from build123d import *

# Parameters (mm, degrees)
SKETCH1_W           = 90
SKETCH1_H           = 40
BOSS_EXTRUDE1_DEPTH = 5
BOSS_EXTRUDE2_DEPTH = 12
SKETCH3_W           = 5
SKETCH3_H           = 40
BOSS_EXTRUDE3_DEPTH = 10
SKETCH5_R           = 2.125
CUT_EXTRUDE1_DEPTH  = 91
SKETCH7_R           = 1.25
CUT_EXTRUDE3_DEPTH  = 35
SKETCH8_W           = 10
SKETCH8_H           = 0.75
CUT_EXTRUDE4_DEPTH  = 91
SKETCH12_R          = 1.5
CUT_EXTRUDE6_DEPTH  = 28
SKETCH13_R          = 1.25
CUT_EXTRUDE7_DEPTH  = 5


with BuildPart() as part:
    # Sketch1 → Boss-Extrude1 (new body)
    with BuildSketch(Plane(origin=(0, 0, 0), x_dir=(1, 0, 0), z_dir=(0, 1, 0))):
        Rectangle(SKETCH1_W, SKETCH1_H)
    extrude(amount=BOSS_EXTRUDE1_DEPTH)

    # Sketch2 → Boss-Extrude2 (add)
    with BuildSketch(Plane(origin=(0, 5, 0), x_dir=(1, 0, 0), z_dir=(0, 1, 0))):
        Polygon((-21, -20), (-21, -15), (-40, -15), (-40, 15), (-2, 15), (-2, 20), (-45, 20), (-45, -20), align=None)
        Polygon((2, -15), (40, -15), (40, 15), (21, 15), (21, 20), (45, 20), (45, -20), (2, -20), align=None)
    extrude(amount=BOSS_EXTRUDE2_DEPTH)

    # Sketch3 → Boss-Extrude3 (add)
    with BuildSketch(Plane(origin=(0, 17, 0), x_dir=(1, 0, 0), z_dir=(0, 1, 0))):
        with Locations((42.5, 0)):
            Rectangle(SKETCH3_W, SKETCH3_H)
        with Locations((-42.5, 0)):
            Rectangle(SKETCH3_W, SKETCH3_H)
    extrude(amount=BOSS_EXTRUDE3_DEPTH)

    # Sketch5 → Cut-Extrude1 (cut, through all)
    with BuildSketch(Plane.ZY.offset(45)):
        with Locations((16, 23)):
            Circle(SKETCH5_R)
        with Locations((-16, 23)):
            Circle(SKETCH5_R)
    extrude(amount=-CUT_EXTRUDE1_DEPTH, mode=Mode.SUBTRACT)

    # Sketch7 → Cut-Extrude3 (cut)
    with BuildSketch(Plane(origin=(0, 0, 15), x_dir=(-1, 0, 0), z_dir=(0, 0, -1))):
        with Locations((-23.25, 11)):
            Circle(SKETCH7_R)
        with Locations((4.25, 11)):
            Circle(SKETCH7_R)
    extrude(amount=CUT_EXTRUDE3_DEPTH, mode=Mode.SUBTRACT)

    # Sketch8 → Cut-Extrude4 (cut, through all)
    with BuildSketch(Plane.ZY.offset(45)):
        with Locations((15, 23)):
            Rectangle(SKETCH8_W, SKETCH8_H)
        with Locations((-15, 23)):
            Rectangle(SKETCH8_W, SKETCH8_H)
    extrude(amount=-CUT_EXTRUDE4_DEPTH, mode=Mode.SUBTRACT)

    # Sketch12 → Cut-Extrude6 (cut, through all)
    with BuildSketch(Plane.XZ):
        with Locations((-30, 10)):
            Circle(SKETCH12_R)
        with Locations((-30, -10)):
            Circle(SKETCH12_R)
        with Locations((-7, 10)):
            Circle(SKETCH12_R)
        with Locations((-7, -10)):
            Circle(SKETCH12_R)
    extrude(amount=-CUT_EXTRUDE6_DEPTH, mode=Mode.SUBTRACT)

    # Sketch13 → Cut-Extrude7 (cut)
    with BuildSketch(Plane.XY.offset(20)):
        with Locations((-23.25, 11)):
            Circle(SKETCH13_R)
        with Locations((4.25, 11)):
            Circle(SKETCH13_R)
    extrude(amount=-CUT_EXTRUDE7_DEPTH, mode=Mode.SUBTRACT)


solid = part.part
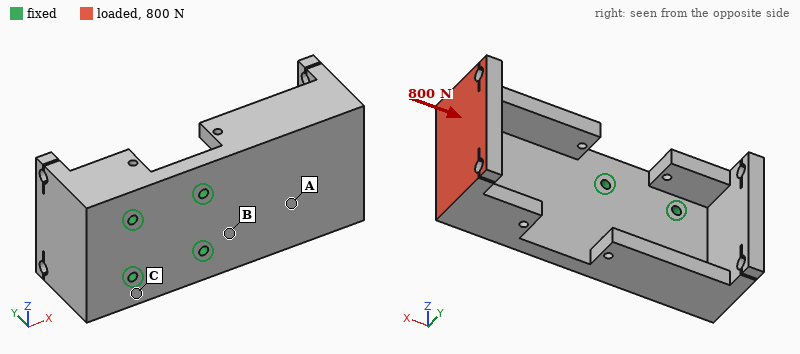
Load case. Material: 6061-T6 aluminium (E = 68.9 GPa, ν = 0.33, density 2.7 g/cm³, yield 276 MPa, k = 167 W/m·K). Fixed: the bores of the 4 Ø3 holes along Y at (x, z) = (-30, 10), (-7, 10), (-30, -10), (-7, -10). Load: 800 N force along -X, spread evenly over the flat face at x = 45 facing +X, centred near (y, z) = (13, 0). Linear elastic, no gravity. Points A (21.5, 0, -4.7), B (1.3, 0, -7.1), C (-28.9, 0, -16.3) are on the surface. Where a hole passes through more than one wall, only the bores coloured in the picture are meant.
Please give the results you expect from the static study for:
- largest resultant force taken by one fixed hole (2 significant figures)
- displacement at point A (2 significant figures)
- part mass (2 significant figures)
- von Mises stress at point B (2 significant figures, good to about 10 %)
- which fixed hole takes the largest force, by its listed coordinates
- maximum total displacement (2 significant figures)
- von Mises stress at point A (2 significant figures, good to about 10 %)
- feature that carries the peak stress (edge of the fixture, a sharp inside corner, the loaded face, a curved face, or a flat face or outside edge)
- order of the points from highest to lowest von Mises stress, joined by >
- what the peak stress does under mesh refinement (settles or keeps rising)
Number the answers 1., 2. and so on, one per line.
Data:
1. 350 N
2. 0.099 mm
3. 89 g
4. 37 MPa
5. (-7, 10)
6. 0.32 mm
7. 16 MPa
8. edge of the fixture
9. B > A > C
10. keeps rising
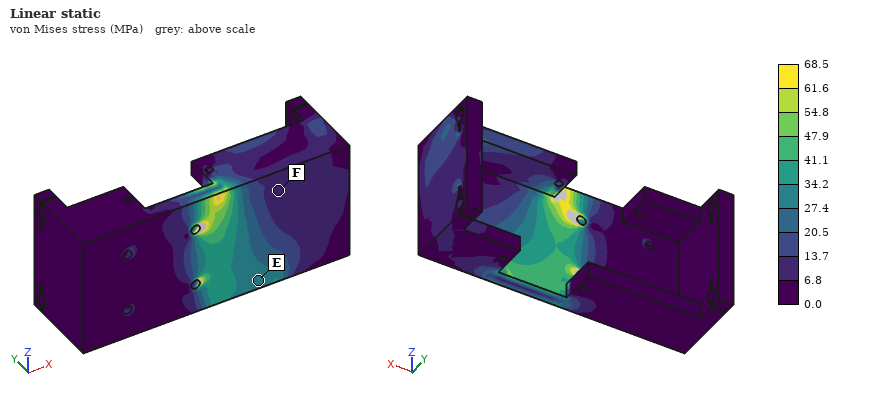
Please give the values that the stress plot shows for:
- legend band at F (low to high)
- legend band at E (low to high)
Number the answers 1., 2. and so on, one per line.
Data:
1. 6.8 to 13.7 MPa
2. 27.4 to 34.2 MPa
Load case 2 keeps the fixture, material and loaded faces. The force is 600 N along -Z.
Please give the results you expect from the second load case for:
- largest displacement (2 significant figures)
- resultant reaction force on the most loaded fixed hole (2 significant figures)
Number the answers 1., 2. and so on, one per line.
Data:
1. 0.14 mm
2. 1.1 kN
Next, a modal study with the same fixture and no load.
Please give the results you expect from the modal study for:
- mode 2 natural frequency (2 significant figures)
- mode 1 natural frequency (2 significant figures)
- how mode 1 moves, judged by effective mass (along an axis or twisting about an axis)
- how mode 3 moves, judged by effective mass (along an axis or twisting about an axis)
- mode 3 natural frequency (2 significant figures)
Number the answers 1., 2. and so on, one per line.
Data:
1. 2400 Hz
2. 950 Hz
3. along Y
4. along Z
5. 5300 Hz
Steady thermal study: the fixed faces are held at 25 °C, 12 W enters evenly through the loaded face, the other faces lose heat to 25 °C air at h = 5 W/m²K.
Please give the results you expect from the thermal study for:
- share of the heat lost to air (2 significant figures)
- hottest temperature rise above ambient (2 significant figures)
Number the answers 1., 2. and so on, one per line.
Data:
1. 3.3 %
2. 18 K
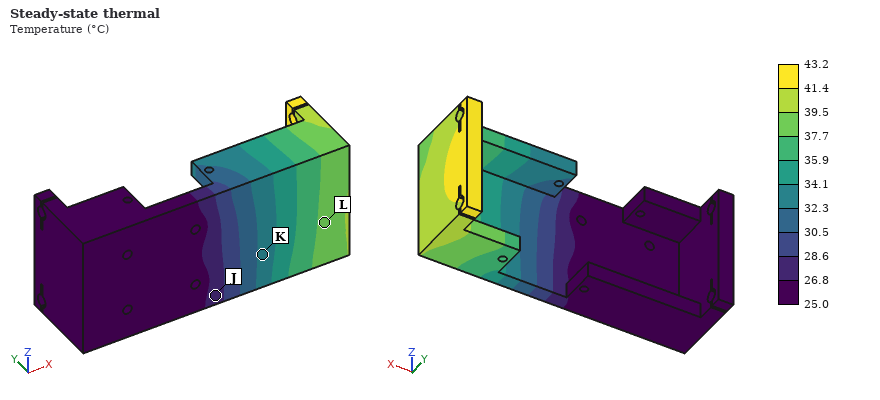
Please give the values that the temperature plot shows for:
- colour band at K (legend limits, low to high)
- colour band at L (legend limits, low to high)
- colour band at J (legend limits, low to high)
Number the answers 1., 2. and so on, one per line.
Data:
1. 32.3 to 34.1 °C
2. 37.7 to 39.5 °C
3. 26.8 to 28.6 °C
